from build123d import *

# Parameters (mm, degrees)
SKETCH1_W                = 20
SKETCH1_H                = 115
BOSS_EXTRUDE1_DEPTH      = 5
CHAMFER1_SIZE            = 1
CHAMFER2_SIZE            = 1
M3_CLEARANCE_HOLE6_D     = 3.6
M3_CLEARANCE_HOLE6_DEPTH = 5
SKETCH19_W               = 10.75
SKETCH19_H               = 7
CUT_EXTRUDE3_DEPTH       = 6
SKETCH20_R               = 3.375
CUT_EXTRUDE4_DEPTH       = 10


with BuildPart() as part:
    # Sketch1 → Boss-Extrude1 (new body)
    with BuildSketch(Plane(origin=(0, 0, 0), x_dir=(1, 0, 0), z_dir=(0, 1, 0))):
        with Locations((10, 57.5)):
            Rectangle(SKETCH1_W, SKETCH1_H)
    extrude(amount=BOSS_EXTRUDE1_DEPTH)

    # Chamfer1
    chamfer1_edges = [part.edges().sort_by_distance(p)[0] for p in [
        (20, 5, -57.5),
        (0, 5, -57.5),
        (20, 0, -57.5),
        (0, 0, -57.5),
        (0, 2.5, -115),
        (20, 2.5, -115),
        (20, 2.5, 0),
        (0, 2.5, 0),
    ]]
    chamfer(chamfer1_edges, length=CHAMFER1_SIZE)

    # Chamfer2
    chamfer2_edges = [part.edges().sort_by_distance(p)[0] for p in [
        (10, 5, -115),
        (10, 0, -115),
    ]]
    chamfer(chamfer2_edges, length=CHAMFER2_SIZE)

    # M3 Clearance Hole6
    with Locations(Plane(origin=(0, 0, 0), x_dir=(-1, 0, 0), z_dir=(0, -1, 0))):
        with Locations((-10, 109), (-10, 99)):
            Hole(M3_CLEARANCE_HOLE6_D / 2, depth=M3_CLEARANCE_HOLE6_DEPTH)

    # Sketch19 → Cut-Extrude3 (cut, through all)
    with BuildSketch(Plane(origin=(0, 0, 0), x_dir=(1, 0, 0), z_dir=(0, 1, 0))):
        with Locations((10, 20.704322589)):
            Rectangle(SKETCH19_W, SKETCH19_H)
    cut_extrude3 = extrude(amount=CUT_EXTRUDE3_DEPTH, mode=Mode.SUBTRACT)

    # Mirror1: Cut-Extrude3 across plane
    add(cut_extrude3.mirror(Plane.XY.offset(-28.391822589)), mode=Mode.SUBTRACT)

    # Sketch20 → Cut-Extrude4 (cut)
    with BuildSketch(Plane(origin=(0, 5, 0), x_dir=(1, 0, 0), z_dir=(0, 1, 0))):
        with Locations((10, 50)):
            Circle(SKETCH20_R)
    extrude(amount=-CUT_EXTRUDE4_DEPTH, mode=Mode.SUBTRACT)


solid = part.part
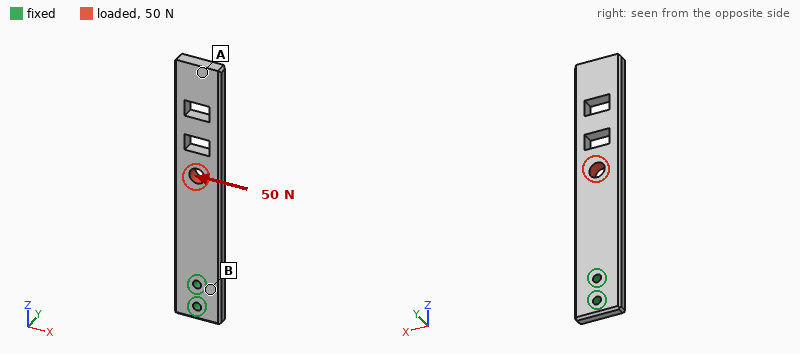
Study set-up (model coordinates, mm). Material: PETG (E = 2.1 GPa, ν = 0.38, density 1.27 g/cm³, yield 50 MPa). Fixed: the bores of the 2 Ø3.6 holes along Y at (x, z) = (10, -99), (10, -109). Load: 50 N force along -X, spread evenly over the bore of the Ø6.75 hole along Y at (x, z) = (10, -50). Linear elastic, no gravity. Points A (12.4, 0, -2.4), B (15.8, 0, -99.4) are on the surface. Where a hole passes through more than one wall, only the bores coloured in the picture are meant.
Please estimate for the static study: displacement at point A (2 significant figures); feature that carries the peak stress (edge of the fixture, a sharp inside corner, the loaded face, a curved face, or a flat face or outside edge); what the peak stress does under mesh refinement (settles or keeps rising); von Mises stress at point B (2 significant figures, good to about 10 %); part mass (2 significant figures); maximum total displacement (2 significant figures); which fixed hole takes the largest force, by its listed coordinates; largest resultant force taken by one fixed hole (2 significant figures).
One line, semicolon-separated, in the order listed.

1.1 mm; edge of the fixture; keeps rising; 4.8 MPa; 13 g; 1.2 mm; (10, -99); 210 N
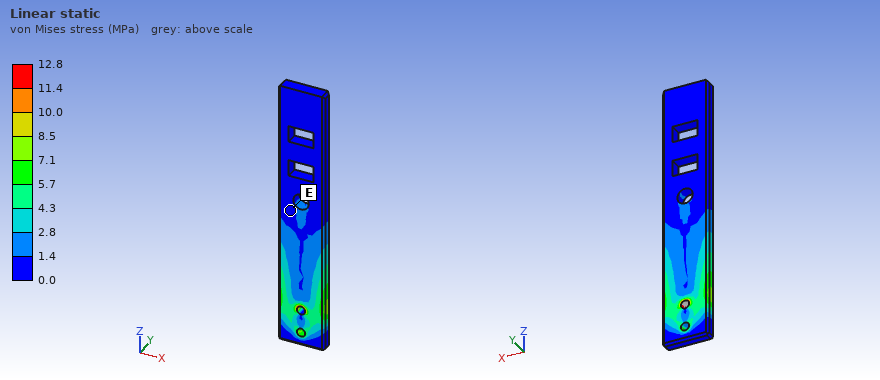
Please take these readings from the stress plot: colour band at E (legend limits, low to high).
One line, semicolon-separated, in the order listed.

0.0 to 1.4 MPa
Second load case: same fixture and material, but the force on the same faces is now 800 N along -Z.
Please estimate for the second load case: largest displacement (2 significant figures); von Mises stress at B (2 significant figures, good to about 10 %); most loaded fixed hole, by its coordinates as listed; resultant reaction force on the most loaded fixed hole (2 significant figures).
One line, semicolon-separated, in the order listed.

0.25 mm; 5.1 MPa; (10, -99); 620 N
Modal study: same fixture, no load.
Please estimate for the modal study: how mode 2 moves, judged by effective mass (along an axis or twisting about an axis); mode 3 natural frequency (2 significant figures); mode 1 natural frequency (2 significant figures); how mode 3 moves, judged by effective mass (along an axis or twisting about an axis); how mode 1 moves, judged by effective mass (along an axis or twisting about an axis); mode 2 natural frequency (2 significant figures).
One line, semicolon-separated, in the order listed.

along X; 580 Hz; 110 Hz; along Y; along Y; 360 Hz
